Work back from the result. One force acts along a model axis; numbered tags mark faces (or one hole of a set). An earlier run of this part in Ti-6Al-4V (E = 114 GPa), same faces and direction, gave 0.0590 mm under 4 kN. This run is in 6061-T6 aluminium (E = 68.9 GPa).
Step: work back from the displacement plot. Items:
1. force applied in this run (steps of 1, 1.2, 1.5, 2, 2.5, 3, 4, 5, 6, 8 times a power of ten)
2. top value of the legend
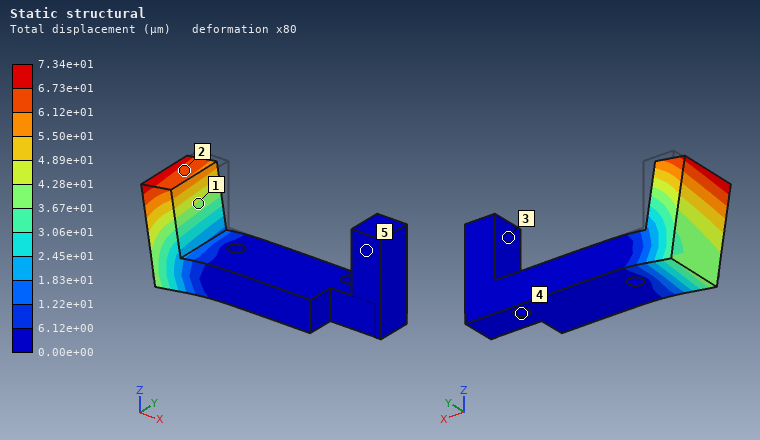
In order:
3 kN
7.34e+01 µm
